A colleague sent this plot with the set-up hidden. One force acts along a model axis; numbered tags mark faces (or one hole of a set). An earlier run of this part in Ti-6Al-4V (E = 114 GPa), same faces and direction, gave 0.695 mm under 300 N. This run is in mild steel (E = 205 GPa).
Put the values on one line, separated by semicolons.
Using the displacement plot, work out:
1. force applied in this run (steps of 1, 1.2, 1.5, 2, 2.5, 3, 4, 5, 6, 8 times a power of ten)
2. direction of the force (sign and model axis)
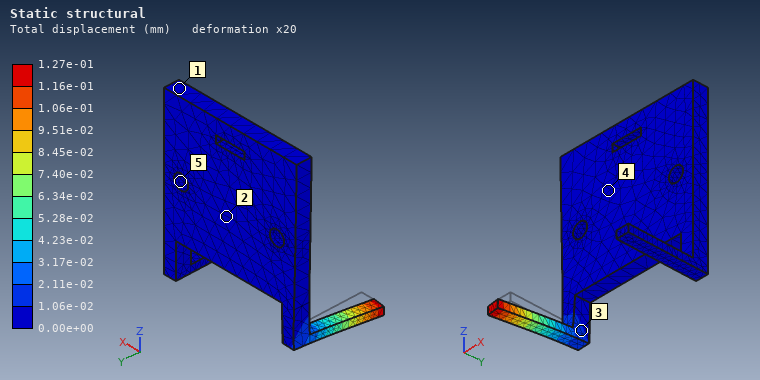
100 N; -X
